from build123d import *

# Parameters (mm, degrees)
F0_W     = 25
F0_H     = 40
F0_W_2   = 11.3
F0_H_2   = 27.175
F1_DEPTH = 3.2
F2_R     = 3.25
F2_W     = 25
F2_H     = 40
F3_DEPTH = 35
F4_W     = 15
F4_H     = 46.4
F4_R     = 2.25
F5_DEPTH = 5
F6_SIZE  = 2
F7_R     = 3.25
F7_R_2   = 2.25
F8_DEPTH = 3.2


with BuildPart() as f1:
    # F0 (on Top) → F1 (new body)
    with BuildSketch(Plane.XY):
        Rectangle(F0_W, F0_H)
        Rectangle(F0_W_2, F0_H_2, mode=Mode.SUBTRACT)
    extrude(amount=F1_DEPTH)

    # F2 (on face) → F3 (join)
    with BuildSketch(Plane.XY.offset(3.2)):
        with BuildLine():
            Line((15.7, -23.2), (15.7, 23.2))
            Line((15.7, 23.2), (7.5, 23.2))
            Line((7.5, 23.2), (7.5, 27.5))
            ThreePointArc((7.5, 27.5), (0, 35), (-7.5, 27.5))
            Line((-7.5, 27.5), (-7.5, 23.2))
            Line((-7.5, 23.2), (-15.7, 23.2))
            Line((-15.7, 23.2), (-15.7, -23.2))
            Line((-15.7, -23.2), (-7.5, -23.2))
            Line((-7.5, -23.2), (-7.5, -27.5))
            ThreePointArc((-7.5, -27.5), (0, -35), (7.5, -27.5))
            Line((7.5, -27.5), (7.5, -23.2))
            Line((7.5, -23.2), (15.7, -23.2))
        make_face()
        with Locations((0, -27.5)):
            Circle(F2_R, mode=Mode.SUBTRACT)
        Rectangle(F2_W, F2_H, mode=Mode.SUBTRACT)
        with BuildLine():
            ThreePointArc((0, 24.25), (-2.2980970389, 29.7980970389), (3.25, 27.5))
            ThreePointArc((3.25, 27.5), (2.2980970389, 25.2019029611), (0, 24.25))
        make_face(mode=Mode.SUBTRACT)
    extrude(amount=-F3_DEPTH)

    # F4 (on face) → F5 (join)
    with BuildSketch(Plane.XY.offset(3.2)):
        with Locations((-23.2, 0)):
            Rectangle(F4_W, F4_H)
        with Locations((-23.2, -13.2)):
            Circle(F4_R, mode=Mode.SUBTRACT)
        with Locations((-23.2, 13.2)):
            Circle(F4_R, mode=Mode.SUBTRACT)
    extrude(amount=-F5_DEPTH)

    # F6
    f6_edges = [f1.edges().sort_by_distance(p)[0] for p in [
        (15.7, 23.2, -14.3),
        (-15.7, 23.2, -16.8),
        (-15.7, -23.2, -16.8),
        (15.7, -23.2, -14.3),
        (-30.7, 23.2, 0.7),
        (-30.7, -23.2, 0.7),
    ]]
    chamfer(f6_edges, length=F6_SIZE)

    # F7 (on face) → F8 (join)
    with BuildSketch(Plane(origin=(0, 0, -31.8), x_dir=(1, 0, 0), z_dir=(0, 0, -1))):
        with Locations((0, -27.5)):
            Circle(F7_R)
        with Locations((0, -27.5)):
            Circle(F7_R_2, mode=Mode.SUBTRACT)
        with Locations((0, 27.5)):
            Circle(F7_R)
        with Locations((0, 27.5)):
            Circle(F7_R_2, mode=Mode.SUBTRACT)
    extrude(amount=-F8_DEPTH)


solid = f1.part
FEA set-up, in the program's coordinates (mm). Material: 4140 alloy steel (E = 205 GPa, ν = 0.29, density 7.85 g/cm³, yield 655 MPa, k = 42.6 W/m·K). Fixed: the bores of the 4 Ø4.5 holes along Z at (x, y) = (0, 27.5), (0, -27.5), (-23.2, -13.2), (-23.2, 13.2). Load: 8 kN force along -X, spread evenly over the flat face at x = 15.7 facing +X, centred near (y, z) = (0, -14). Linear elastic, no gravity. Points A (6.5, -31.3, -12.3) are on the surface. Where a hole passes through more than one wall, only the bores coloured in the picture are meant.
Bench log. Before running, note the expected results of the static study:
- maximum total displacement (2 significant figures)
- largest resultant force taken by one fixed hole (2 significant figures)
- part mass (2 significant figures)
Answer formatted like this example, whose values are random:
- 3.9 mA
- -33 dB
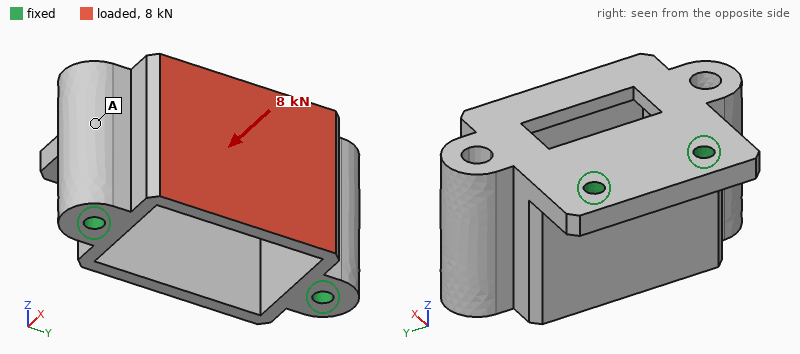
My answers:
- 0.12 mm
- 2.6 kN
- 230 g
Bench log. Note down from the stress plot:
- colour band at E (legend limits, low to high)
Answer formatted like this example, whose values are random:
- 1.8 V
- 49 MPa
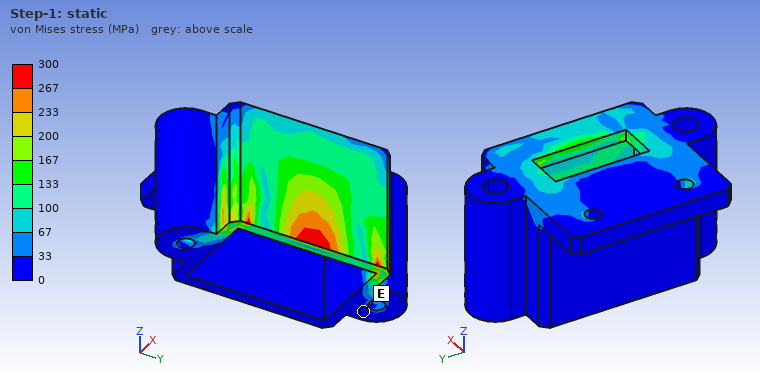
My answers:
- 0 to 33 MPa
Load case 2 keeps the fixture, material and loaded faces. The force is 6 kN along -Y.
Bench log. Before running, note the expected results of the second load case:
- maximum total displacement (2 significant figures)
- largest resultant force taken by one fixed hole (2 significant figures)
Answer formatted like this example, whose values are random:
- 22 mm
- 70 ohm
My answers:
- 49 µm
- 2.4 kN
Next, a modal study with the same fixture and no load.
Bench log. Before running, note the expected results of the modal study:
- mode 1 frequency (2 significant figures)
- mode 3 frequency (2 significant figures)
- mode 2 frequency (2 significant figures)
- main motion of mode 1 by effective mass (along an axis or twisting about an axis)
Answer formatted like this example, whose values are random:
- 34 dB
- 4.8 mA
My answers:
- 7600 Hz
- 9200 Hz
- 8600 Hz
- along Y
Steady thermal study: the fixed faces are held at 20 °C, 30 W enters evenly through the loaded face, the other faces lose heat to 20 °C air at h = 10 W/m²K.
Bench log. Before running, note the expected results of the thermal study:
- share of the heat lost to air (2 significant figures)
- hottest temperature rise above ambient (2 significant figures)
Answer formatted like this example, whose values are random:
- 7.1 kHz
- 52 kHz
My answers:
- 11 %
- 72 K
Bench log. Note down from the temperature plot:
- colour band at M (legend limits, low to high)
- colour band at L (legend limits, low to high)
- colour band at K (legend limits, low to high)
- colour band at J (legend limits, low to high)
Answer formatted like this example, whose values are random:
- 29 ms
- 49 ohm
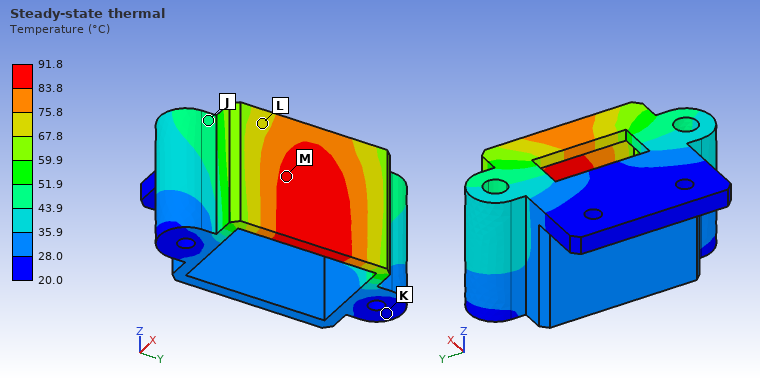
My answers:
- 83.8 to 91.8 °C
- 67.8 to 75.8 °C
- 20.0 to 28.0 °C
- 43.9 to 51.9 °C
